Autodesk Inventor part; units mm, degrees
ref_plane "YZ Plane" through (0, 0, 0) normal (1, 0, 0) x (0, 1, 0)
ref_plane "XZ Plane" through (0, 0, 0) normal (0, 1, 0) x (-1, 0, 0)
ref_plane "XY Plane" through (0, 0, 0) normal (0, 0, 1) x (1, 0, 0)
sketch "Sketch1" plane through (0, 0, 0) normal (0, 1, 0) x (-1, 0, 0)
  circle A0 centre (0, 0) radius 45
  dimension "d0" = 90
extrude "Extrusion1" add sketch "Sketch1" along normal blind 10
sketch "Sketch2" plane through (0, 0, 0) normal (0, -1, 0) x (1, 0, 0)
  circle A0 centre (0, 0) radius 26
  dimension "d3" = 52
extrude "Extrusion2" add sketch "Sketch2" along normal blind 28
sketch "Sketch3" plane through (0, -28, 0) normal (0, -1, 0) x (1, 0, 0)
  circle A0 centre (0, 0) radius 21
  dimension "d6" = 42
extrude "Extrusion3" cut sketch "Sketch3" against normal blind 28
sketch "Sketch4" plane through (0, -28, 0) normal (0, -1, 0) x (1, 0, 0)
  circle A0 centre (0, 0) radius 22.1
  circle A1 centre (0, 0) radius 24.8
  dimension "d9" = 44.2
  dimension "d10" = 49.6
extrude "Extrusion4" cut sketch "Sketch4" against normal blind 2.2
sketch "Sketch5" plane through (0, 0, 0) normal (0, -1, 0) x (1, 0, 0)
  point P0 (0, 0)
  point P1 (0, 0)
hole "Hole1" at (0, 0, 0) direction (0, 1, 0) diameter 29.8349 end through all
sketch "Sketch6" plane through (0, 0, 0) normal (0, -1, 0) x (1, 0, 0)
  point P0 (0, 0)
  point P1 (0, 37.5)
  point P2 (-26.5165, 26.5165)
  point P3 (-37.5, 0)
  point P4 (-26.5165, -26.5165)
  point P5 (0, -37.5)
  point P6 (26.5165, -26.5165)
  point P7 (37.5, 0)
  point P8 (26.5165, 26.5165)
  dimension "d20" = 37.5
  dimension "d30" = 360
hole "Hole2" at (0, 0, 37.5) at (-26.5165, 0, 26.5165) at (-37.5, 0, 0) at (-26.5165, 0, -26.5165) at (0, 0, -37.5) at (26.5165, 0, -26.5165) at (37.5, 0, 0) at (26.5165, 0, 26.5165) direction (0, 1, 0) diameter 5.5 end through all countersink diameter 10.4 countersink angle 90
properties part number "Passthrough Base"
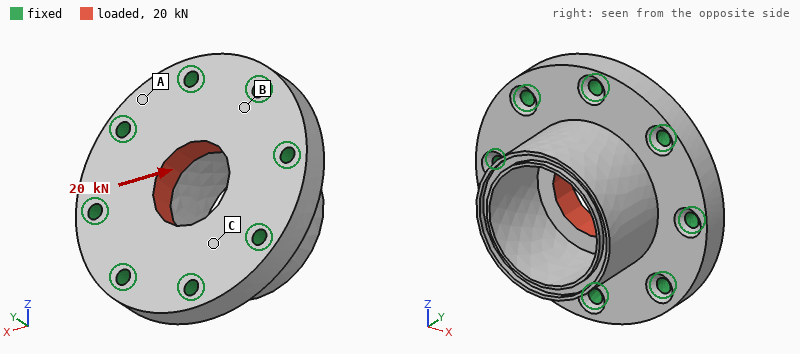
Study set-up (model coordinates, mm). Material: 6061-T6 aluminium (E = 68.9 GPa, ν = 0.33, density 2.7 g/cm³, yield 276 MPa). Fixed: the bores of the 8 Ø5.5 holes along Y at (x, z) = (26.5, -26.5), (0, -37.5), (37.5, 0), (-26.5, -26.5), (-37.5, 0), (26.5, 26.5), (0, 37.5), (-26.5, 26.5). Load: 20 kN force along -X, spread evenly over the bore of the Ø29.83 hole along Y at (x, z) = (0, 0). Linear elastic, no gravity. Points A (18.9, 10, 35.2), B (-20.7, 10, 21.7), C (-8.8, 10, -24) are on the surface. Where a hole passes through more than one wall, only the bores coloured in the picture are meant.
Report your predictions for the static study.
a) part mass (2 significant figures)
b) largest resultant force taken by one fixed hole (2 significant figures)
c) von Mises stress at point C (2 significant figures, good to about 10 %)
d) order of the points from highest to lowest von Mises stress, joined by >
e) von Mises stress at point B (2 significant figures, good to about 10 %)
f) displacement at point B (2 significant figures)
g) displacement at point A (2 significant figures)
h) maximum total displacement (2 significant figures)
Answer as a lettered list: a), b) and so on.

a) 200 g
b) 3.9 kN
c) 13 MPa
d) B > C > A
e) 24 MPa
f) 2.0 µm
g) 1.3 µm
h) 8.1 µm
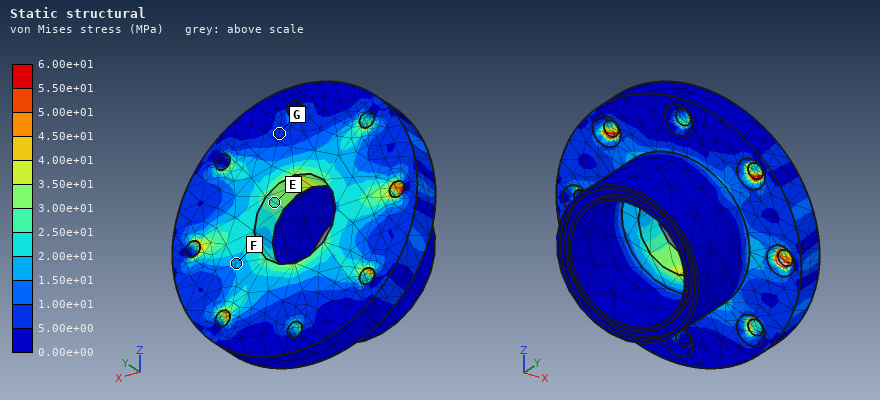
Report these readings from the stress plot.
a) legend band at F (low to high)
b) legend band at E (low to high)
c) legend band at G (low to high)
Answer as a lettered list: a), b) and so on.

a) 1.50e+01 to 2.00e+01 MPa
b) 2.50e+01 to 3.00e+01 MPa
c) 5.00e+00 to 1.00e+01 MPa
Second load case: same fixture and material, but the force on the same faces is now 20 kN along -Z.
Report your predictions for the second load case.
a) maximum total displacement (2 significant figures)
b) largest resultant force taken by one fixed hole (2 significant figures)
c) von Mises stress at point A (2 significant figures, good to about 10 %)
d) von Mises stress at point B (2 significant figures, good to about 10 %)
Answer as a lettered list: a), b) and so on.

a) 8.1 µm
b) 3.9 kN
c) 6.5 MPa
d) 23 MPa
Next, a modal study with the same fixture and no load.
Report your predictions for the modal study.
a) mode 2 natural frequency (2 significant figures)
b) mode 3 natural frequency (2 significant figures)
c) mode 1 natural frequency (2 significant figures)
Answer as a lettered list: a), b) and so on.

a) 12 kHz
b) 14 kHz
c) 12 kHz
